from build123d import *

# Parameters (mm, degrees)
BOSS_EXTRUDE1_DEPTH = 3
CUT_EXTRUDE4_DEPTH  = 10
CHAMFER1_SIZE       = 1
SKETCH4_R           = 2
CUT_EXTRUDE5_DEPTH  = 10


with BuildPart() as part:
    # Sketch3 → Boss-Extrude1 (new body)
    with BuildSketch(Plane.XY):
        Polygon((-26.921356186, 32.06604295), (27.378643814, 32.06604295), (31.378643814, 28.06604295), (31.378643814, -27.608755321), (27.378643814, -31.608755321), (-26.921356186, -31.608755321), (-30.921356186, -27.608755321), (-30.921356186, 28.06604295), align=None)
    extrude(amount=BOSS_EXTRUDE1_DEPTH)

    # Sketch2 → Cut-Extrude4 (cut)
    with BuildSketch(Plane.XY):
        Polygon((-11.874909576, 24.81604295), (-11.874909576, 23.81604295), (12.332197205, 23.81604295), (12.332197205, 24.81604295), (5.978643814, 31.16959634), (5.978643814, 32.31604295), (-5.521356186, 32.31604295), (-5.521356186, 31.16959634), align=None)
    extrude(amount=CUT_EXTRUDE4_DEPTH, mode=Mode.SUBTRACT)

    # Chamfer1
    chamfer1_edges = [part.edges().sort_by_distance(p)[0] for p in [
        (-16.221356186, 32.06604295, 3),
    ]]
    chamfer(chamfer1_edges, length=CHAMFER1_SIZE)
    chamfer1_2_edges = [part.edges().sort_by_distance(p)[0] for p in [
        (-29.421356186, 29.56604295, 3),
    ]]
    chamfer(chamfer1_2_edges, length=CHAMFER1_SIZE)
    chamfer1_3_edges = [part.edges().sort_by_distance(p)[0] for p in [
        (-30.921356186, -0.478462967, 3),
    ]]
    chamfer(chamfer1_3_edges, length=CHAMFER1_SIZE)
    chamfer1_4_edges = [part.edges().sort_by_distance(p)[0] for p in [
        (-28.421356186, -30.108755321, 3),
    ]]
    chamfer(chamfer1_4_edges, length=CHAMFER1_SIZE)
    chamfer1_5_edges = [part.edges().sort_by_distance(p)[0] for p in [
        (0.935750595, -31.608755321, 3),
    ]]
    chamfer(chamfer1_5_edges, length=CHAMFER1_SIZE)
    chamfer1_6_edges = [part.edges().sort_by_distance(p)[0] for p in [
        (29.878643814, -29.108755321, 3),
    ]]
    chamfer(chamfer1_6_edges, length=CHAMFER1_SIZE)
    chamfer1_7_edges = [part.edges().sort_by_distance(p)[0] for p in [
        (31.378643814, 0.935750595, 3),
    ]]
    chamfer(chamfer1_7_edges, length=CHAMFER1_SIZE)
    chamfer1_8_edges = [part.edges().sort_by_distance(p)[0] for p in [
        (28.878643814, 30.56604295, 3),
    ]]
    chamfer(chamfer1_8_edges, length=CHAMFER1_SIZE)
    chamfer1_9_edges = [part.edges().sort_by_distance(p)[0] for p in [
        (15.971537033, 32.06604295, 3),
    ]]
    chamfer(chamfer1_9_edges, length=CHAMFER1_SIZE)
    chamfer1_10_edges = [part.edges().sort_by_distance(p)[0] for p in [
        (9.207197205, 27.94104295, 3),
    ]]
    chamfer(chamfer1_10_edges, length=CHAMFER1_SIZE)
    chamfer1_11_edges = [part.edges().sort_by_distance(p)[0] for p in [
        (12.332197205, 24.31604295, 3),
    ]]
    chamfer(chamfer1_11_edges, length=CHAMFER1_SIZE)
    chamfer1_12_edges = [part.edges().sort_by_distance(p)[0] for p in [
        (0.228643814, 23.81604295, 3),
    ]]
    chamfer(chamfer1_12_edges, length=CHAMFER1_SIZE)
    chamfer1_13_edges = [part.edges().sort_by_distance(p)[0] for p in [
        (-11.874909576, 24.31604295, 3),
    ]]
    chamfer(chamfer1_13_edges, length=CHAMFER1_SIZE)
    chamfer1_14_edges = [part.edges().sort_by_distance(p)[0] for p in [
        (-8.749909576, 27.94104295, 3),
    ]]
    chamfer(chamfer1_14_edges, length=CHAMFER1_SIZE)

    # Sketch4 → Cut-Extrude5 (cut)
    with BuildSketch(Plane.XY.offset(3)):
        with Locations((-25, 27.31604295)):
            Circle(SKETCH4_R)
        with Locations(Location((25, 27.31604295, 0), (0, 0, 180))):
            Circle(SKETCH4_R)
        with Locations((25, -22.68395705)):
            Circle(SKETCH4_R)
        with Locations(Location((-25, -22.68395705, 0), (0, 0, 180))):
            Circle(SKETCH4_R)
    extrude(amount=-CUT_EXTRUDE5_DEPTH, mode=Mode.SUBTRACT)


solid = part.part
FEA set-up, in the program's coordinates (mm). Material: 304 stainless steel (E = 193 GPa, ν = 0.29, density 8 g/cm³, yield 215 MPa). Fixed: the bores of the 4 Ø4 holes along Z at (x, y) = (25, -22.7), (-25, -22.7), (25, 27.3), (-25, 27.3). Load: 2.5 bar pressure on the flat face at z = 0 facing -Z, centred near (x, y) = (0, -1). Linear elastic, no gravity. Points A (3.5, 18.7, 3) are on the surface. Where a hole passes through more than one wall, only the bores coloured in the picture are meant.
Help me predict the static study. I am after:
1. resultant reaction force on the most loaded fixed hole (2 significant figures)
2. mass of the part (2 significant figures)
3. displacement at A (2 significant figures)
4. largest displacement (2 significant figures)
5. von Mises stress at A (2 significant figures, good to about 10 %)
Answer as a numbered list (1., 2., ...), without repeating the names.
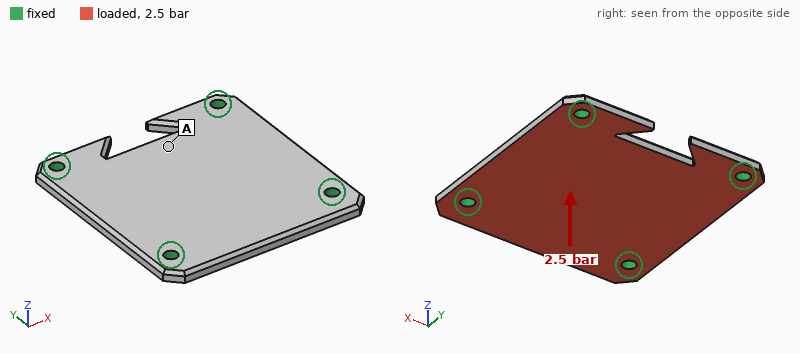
1. 260 N
2. 89 g
3. 17 µm
4. 23 µm
5. 21 MPa
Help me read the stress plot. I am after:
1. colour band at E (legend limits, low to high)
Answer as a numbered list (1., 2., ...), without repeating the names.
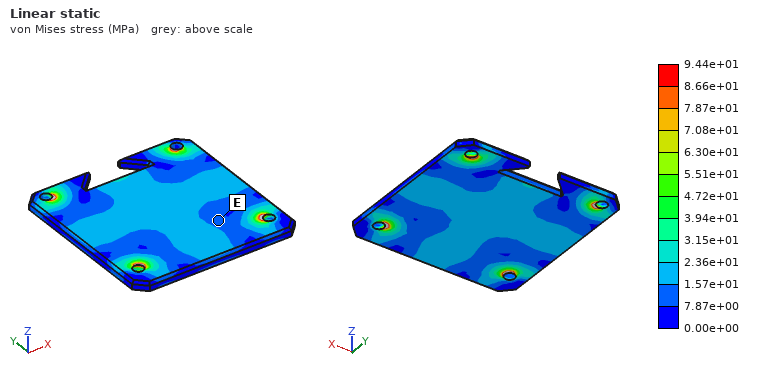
1. 7.87e+00 to 1.57e+01 MPa
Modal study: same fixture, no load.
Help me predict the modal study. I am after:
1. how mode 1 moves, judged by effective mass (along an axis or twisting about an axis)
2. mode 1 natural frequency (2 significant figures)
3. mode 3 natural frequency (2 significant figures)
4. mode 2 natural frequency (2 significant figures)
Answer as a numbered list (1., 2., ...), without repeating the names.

1. along Z
2. 4100 Hz
3. 6800 Hz
4. 6700 Hz
